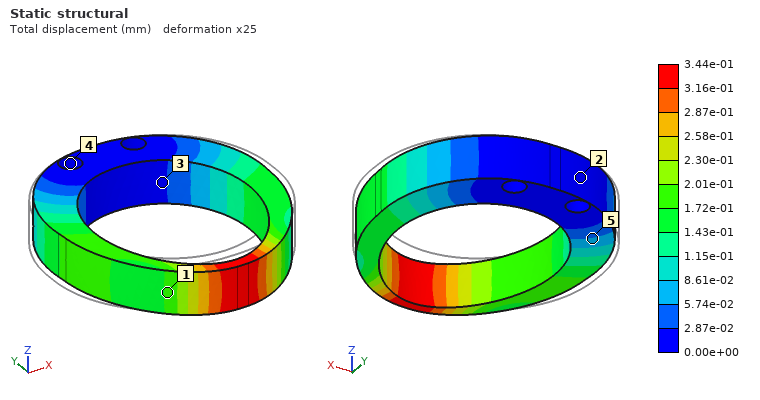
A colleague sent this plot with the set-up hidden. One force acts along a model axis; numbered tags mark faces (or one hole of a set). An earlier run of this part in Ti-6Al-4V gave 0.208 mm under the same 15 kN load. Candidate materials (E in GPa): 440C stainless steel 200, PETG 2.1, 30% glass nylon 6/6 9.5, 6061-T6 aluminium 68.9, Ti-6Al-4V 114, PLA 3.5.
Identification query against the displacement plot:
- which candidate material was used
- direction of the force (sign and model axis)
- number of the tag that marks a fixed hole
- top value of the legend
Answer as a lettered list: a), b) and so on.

a) 6061-T6 aluminium
b) -Y
c) 4
d) 3.44e-01 mm
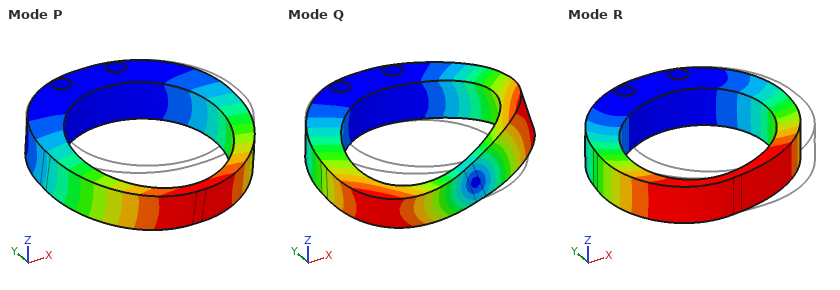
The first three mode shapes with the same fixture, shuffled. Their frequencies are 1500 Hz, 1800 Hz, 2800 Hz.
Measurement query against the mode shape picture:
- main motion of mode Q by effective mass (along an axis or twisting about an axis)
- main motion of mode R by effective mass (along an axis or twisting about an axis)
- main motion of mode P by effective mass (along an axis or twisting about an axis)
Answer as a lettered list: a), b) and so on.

a) twisting about Y
b) along X
c) along Z
